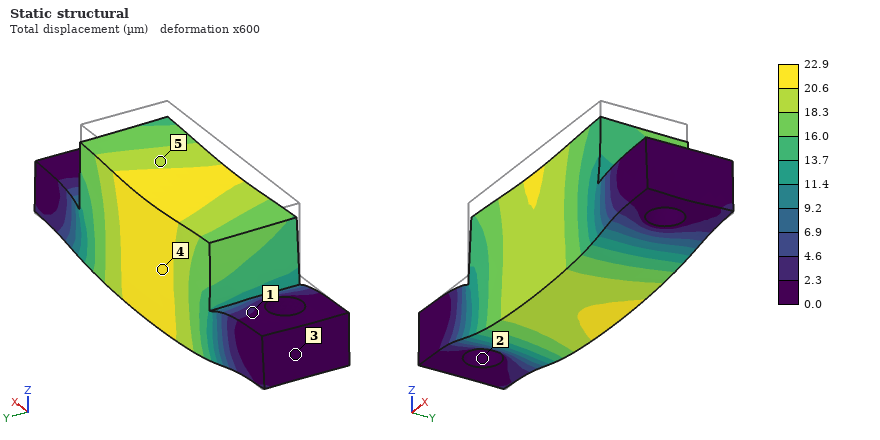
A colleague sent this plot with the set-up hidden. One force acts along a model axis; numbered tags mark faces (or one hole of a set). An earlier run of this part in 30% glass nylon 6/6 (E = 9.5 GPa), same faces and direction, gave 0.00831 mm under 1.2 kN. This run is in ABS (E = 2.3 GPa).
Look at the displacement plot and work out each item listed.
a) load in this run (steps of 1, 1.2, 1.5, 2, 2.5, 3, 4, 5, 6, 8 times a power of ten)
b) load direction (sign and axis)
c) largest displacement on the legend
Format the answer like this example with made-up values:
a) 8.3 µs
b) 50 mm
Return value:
a) 800 N
b) -Z
c) 22.9 µm
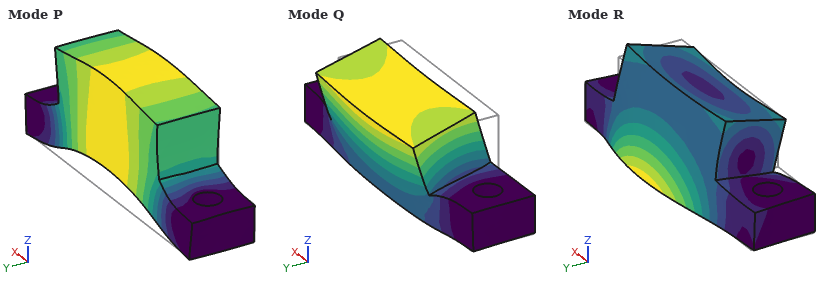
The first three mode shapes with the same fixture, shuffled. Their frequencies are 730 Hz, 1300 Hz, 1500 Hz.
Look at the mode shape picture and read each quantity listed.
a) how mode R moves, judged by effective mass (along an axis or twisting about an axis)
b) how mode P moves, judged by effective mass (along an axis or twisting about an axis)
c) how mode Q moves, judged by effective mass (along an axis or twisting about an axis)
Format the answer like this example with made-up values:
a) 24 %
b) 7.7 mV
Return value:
a) along Y
b) along Z
c) along Y
